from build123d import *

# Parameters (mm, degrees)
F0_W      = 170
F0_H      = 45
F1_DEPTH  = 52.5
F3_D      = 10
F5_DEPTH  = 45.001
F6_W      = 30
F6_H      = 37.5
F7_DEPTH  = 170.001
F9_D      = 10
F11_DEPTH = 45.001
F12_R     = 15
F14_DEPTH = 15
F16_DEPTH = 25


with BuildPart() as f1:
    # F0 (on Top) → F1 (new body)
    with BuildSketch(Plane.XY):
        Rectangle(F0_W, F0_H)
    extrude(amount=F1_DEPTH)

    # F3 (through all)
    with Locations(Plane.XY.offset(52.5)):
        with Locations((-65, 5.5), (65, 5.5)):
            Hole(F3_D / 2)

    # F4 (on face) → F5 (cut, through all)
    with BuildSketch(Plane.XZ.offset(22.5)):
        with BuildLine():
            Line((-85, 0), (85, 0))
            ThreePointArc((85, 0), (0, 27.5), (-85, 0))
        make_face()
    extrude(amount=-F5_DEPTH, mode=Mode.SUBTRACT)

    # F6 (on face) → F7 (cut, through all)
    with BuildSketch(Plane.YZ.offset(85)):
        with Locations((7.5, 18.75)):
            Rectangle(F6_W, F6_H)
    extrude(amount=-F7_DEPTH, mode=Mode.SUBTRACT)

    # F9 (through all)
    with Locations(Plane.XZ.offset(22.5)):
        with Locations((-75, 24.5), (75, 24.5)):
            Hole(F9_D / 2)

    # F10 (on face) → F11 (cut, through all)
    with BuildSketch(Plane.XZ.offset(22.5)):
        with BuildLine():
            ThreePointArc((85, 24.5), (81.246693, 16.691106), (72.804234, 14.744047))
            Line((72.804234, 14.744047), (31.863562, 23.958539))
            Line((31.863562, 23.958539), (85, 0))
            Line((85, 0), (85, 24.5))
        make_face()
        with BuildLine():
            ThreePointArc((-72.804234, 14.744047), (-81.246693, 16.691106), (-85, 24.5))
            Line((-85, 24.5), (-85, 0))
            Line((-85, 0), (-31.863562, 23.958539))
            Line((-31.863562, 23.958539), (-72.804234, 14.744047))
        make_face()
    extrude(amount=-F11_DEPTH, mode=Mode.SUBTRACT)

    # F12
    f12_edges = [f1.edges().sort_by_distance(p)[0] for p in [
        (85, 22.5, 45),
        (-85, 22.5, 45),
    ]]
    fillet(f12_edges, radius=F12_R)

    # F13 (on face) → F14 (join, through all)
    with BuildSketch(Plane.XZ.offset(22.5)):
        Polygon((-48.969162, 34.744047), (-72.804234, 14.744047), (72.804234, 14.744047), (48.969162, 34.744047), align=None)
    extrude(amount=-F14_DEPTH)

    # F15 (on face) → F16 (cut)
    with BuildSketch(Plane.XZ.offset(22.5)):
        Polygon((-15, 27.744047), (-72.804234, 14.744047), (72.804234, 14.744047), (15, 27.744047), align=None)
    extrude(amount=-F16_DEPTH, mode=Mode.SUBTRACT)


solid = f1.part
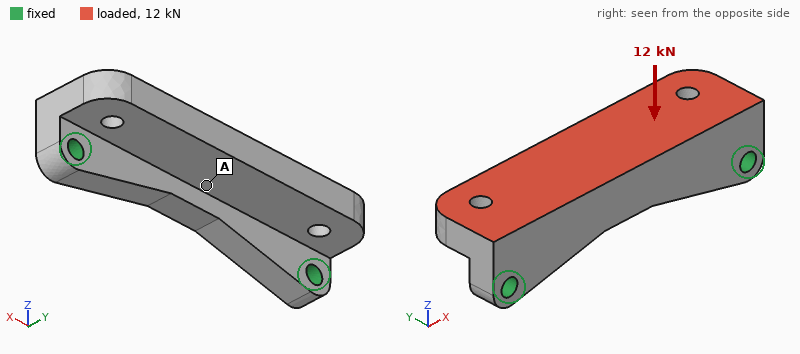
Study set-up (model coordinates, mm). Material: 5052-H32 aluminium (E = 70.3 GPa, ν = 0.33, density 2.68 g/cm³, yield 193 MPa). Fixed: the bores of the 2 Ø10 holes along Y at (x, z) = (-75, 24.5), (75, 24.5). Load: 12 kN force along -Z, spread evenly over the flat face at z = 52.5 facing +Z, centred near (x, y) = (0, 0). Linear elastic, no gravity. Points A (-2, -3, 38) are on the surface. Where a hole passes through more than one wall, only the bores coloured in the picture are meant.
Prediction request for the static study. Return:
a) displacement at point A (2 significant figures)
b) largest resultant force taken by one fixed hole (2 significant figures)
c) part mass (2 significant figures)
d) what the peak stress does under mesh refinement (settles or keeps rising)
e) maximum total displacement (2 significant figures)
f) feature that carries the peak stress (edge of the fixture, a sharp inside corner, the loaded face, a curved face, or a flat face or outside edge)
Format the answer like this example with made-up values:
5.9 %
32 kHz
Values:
0.098 mm
7.8 kN
400 g
keeps rising
0.20 mm
edge of the fixture
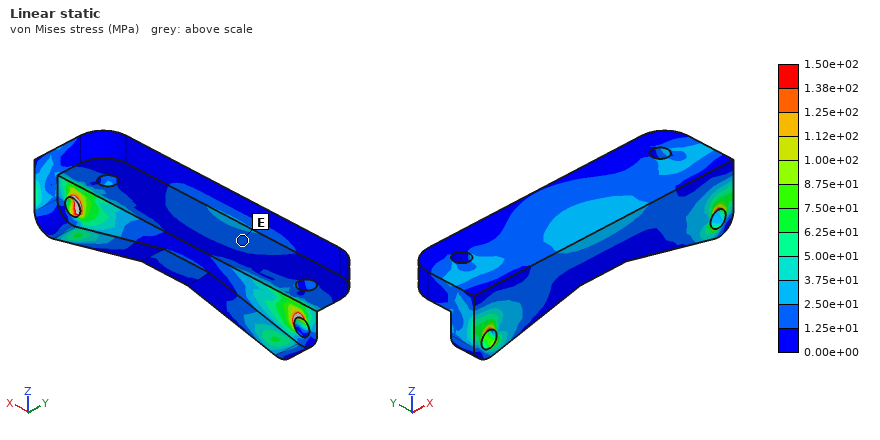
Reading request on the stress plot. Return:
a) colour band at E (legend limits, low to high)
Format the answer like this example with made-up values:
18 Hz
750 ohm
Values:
1.25e+01 to 2.50e+01 MPa
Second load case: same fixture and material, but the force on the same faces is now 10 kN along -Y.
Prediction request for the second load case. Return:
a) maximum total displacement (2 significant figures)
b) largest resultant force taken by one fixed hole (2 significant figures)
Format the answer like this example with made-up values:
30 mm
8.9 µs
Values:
0.18 mm
5.1 kN
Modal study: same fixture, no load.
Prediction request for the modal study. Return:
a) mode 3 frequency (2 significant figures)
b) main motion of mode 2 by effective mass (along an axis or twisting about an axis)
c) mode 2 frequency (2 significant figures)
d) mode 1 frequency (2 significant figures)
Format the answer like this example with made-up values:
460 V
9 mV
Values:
5300 Hz
along Y
5000 Hz
2600 Hz
